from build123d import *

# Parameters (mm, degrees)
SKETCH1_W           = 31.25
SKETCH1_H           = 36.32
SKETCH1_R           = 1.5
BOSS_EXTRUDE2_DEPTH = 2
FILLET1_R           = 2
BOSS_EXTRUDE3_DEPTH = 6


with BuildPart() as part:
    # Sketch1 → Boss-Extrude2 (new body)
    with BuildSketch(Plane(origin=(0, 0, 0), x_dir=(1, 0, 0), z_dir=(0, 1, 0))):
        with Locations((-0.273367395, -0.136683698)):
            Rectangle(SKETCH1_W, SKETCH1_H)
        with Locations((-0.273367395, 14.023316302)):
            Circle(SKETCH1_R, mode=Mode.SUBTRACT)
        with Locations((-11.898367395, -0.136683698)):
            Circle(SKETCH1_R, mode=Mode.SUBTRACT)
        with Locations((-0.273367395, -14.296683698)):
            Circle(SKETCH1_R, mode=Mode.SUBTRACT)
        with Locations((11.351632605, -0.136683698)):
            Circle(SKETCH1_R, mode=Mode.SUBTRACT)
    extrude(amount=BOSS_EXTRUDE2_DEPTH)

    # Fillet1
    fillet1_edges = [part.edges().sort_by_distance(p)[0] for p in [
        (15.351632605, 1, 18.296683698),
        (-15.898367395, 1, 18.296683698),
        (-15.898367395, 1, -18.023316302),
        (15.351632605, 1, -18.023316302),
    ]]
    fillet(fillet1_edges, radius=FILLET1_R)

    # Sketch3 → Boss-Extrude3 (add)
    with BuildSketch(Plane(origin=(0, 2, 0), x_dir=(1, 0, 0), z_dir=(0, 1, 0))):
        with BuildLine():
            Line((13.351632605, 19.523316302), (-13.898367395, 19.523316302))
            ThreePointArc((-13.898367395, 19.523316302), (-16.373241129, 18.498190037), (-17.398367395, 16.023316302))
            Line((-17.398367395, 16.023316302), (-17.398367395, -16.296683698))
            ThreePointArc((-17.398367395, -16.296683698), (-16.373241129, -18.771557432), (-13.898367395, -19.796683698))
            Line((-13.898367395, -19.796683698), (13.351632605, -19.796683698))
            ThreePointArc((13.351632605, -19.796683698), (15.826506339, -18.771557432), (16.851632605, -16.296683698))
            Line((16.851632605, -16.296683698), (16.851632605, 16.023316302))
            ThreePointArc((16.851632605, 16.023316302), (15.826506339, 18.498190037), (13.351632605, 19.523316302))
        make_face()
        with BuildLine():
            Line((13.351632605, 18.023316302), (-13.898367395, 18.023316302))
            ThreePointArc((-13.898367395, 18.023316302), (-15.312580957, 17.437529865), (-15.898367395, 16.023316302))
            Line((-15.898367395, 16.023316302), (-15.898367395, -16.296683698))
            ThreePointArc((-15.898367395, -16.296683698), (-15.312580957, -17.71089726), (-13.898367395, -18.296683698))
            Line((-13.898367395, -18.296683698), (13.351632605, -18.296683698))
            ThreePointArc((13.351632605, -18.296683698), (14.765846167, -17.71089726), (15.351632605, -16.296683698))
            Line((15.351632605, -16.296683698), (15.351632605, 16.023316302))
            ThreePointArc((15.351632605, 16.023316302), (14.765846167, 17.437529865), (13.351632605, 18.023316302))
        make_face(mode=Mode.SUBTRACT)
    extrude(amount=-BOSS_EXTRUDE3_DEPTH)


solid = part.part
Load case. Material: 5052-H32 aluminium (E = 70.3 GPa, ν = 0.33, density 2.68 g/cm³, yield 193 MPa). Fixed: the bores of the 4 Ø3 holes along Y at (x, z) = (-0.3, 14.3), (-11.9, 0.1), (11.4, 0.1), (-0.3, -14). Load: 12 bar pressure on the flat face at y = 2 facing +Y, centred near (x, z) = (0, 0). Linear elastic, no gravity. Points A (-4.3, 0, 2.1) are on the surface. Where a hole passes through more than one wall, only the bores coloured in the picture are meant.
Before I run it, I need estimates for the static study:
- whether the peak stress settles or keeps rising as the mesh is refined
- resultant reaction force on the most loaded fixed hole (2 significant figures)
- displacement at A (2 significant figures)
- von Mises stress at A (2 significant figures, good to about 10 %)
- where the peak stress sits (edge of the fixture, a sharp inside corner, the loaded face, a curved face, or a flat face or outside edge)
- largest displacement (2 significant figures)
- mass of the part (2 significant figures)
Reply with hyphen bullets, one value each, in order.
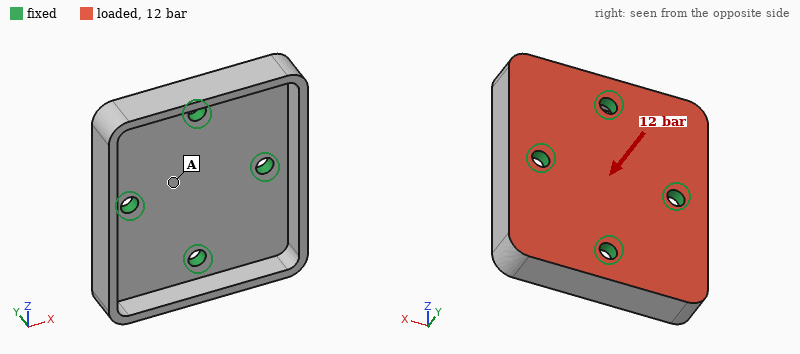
- keeps rising
- 400 N
- 8.0 µm
- 15 MPa
- edge of the fixture
- 20 µm
- 9.2 g
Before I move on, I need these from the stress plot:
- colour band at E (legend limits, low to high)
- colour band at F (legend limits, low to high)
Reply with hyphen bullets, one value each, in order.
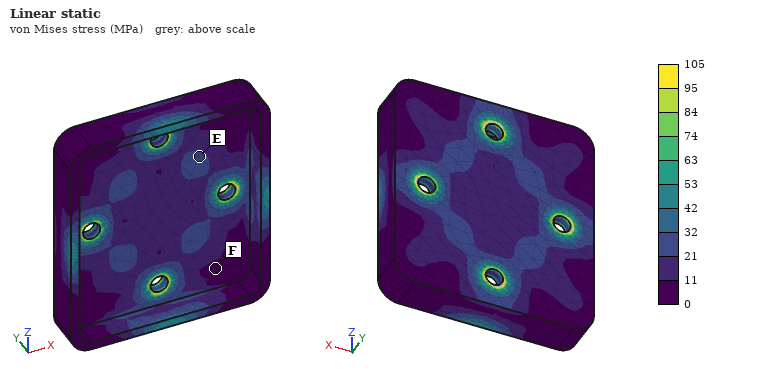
- 21 to 32 MPa
- 0 to 11 MPa
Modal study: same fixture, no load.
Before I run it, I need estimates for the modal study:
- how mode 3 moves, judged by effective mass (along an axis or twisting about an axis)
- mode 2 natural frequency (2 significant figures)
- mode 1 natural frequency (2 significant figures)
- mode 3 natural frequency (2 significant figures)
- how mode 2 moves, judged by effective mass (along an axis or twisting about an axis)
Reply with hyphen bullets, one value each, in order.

- twisting about X
- 12 kHz
- 8100 Hz
- 13 kHz
- twisting about Z
